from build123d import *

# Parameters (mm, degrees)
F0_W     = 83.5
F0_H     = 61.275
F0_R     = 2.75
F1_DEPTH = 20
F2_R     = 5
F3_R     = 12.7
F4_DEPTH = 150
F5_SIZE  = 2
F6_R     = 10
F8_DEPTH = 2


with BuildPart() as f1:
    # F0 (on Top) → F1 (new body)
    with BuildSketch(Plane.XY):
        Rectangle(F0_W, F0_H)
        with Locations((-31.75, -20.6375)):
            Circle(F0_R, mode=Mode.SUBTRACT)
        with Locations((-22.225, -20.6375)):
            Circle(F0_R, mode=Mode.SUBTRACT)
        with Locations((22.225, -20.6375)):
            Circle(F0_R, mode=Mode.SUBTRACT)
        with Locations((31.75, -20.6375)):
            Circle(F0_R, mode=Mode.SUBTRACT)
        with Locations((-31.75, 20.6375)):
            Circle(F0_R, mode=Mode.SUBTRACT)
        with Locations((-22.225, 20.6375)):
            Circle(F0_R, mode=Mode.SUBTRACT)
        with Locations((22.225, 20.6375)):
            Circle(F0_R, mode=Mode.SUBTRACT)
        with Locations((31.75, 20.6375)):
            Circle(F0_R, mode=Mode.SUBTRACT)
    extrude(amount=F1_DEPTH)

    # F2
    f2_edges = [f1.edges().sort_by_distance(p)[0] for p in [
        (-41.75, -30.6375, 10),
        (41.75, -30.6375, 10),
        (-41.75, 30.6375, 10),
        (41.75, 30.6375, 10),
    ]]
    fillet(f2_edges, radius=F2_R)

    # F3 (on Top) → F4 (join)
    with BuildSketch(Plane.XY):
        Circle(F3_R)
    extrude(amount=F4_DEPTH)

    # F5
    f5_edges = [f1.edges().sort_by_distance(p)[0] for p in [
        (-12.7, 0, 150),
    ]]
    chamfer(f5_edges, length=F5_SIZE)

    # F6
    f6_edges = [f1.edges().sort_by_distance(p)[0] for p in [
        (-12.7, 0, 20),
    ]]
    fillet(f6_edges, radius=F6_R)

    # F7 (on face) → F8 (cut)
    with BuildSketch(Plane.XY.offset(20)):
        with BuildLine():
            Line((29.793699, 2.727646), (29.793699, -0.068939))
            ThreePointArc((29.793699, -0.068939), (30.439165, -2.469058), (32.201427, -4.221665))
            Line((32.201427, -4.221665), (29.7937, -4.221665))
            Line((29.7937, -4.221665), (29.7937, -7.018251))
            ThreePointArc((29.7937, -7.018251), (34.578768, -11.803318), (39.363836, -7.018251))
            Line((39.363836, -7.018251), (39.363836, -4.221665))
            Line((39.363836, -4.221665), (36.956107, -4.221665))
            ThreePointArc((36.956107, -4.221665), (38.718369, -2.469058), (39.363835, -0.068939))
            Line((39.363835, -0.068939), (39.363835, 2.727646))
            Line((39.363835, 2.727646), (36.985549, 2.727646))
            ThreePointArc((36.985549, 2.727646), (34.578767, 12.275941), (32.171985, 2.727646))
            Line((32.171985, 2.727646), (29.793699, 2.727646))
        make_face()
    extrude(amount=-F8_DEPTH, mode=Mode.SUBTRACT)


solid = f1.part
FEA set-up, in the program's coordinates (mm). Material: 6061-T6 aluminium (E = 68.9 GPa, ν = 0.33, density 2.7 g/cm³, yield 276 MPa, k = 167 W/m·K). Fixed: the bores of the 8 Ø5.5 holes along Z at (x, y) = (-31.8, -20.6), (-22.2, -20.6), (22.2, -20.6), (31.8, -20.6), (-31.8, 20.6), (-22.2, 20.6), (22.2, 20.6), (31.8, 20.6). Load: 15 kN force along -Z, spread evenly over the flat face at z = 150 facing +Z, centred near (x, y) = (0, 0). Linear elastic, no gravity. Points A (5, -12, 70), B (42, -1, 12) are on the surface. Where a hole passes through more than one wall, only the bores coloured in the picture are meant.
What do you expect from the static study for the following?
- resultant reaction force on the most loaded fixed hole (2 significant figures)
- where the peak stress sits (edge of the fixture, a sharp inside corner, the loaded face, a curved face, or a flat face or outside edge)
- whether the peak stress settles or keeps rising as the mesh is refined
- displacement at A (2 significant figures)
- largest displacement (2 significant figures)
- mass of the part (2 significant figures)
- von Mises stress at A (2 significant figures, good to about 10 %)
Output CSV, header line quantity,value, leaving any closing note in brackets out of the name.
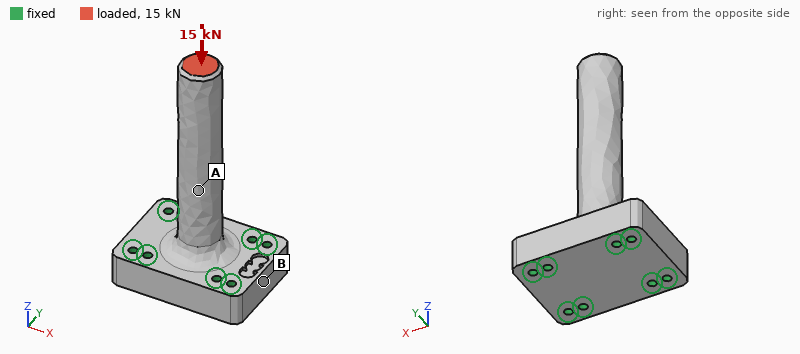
quantity,value
resultant reaction force on the most loaded fixed hole,3.4 kN
where the peak stress sits,edge of the fixture
whether the peak stress settles or keeps rising as the mesh is refined,keeps rising
displacement at A,29 µm
largest displacement,65 µm
mass of the part,450 g
von Mises stress at A,29 MPa
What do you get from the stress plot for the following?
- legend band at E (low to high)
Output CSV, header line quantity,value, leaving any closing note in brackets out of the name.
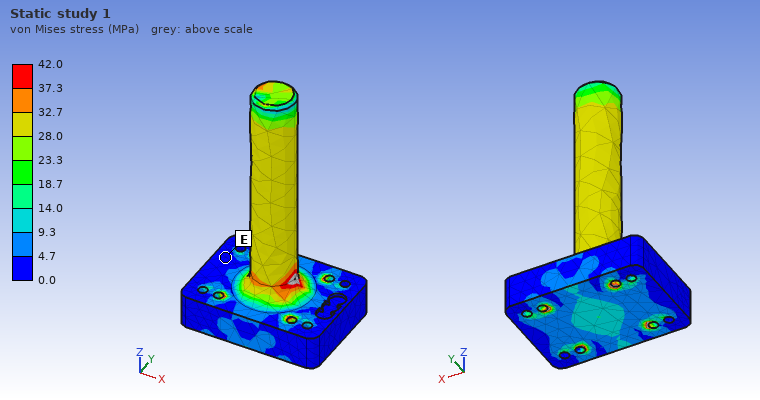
quantity,value
legend band at E,0.0 to 4.7 MPa
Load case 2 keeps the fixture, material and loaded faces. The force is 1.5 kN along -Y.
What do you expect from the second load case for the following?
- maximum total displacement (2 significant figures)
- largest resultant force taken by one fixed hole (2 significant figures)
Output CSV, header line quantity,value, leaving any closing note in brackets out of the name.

quantity,value
maximum total displacement,0.81 mm
largest resultant force taken by one fixed hole,2.3 kN
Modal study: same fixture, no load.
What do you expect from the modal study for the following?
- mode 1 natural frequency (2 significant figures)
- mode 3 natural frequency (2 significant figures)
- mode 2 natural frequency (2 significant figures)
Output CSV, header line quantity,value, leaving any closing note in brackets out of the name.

quantity,value
mode 1 natural frequency,1000 Hz
mode 3 natural frequency,5800 Hz
mode 2 natural frequency,1000 Hz
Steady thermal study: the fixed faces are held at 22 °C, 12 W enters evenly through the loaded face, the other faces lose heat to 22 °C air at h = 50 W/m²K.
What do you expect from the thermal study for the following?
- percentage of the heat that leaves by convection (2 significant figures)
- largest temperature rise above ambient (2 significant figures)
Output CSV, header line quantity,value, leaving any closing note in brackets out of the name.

quantity,value
percentage of the heat that leaves by convection,33 %
largest temperature rise above ambient,15 K
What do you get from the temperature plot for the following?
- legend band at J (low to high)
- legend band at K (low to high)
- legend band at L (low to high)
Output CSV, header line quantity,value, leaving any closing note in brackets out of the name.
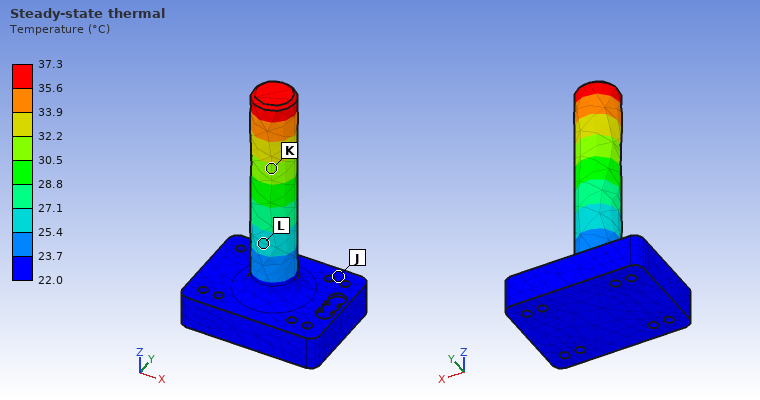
quantity,value
legend band at J,22.0 to 23.7 °C
legend band at K,30.5 to 32.2 °C
legend band at L,25.4 to 27.1 °C
